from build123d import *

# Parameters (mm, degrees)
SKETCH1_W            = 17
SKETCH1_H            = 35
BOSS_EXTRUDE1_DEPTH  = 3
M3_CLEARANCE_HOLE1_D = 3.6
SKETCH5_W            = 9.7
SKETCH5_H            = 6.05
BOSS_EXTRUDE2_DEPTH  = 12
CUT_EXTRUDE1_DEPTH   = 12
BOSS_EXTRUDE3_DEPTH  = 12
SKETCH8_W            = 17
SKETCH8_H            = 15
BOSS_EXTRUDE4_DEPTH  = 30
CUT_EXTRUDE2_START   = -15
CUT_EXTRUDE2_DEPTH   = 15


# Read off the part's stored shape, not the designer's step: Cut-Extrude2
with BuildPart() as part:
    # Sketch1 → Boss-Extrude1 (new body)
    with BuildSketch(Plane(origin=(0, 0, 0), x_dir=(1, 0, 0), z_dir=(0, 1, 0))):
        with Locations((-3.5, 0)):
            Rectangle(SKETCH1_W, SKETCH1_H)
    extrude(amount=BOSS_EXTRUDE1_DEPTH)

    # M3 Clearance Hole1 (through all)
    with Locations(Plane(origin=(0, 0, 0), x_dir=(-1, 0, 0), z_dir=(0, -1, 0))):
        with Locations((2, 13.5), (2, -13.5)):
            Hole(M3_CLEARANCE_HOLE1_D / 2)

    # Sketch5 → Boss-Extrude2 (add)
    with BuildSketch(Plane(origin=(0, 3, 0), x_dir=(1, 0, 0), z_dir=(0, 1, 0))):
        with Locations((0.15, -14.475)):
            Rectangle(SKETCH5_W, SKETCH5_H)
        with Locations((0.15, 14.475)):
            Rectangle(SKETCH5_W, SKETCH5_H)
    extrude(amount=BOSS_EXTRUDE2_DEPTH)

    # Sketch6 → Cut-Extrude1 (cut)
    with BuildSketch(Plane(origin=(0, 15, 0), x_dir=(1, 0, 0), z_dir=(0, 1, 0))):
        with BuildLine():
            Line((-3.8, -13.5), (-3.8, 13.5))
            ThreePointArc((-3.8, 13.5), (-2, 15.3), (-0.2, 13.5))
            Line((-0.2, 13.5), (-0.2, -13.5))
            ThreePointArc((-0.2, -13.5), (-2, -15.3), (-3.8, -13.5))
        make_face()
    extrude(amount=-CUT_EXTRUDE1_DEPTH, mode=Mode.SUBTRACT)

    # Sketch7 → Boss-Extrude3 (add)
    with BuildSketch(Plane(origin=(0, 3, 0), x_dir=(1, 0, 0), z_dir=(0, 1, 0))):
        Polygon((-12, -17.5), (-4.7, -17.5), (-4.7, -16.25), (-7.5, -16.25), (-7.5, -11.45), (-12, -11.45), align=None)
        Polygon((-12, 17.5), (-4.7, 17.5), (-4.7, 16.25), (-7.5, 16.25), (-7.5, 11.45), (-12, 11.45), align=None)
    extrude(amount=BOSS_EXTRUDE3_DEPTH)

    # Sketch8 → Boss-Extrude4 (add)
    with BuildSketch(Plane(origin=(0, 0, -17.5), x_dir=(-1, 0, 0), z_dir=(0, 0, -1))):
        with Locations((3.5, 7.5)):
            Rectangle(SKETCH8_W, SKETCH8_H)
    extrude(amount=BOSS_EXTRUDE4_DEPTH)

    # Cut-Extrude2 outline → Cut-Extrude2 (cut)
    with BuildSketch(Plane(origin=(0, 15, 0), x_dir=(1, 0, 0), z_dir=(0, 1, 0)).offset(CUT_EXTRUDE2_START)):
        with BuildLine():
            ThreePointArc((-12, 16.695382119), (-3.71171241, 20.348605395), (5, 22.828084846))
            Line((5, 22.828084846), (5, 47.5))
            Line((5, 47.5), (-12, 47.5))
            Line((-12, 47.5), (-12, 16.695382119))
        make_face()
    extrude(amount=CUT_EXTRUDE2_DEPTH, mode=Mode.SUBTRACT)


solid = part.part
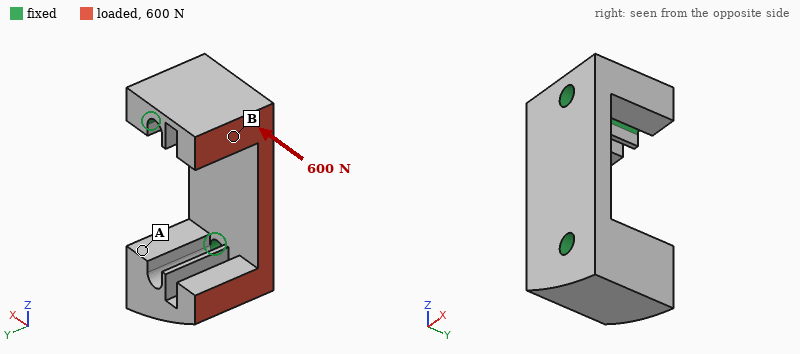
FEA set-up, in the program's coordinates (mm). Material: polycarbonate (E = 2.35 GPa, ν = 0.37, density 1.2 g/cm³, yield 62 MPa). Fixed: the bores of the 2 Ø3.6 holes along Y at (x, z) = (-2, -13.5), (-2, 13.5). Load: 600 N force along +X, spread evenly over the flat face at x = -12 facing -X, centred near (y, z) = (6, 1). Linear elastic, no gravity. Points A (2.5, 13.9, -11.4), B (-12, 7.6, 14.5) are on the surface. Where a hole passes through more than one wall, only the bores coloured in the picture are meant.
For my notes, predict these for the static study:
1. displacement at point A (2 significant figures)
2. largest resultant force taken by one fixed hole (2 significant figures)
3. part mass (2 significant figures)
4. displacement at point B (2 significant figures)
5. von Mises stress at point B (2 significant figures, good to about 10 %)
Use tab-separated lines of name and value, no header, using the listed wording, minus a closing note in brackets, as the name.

displacement at point A	0.24 mm
largest resultant force taken by one fixed hole	310 N
part mass	5.1 g
displacement at point B	0.11 mm
von Mises stress at point B	12 MPa
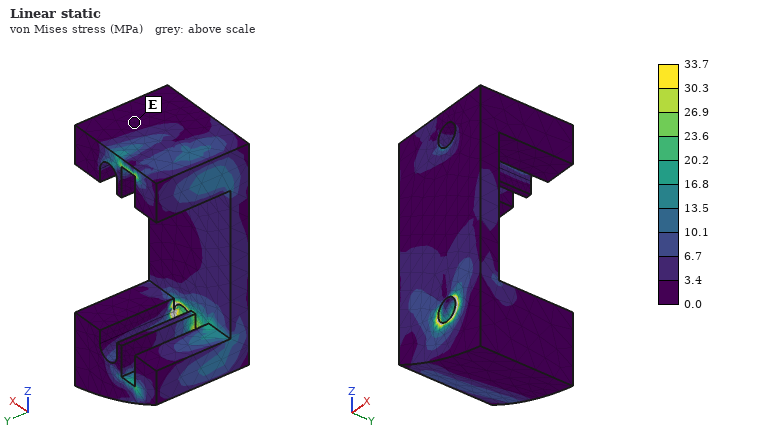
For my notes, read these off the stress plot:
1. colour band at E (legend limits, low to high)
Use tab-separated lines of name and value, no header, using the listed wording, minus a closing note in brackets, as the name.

colour band at E	0.0 to 3.4 MPa
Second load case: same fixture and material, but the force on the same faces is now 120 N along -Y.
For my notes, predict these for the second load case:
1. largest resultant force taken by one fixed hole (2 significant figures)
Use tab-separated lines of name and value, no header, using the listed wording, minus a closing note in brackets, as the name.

largest resultant force taken by one fixed hole	64 N
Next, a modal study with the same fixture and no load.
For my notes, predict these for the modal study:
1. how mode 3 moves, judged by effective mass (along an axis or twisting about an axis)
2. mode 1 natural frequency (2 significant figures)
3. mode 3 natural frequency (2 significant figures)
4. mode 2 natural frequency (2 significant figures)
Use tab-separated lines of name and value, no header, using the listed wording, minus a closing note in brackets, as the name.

how mode 3 moves, judged by effective mass	along Y
mode 1 natural frequency	3100 Hz
mode 3 natural frequency	5500 Hz
mode 2 natural frequency	3400 Hz
